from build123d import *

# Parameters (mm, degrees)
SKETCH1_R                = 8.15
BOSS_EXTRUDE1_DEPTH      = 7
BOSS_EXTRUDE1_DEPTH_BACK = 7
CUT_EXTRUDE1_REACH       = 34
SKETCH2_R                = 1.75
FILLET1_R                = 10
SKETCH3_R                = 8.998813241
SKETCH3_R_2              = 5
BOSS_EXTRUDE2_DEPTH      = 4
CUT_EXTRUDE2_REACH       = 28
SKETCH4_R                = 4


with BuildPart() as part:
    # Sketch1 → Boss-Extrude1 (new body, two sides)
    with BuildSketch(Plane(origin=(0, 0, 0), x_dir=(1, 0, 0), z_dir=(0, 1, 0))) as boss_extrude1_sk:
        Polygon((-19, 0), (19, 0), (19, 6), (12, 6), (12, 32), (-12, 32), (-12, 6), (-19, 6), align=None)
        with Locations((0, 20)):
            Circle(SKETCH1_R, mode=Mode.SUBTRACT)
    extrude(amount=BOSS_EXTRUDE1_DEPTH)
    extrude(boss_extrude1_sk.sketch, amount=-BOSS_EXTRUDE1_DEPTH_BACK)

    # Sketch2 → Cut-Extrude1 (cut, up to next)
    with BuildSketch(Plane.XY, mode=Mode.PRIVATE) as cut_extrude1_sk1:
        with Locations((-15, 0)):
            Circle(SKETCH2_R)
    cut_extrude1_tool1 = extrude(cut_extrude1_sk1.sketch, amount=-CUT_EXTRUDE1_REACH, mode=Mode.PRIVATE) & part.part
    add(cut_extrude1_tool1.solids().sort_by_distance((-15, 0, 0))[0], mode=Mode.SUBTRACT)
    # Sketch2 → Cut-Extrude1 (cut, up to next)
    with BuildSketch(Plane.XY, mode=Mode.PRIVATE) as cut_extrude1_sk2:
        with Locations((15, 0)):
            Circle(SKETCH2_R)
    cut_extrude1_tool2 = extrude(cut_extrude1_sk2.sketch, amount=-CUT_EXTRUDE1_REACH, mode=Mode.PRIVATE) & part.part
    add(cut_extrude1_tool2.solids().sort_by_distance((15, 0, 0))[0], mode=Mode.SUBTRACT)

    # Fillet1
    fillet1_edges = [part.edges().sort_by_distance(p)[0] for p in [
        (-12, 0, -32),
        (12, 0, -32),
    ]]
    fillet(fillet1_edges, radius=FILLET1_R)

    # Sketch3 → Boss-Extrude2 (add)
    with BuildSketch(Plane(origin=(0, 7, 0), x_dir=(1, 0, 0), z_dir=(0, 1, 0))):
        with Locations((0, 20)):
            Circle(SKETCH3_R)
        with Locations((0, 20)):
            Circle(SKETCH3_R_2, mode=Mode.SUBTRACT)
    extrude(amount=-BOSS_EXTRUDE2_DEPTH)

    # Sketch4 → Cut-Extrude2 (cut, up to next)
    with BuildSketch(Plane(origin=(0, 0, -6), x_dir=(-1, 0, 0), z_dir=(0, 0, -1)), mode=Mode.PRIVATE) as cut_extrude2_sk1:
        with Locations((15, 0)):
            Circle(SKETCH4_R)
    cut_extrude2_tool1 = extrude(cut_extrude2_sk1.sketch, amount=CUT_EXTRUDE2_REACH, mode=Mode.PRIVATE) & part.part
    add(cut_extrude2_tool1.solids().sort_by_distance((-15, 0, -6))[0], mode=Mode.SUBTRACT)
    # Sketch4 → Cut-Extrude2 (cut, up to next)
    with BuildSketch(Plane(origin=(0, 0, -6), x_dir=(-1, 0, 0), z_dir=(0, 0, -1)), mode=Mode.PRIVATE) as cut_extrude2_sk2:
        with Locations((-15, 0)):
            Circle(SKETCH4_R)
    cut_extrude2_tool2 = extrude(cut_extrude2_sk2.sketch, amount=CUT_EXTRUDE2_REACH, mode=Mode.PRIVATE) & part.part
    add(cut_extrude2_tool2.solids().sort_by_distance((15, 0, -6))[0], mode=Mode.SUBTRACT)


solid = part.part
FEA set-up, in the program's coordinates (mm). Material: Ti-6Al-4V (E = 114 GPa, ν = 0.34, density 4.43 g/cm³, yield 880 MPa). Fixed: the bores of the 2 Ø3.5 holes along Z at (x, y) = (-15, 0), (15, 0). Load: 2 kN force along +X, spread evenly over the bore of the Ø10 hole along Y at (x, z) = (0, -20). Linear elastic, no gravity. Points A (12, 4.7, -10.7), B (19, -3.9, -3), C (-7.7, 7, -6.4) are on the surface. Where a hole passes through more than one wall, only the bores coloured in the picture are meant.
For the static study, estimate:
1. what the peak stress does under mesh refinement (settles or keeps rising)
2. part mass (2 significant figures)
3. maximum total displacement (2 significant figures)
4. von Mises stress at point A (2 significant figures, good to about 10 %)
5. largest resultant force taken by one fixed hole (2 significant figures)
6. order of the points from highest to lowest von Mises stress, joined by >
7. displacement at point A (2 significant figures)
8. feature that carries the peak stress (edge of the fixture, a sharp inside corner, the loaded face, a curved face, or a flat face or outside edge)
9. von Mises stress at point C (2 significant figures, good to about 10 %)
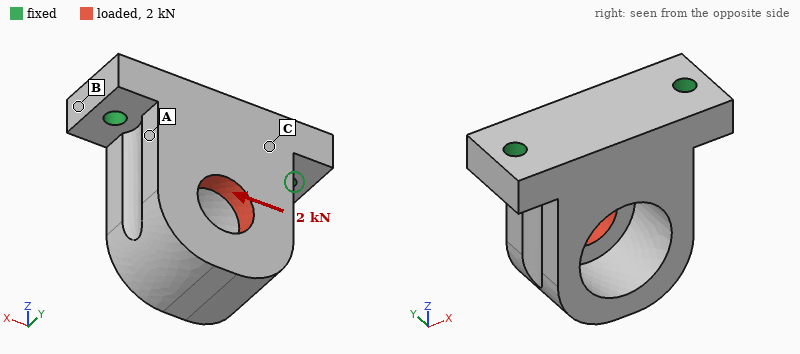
keeps rising
38 g
20 µm
35 MPa
1.7 kN
A > C > B
6.1 µm
edge of the fixture
21 MPa
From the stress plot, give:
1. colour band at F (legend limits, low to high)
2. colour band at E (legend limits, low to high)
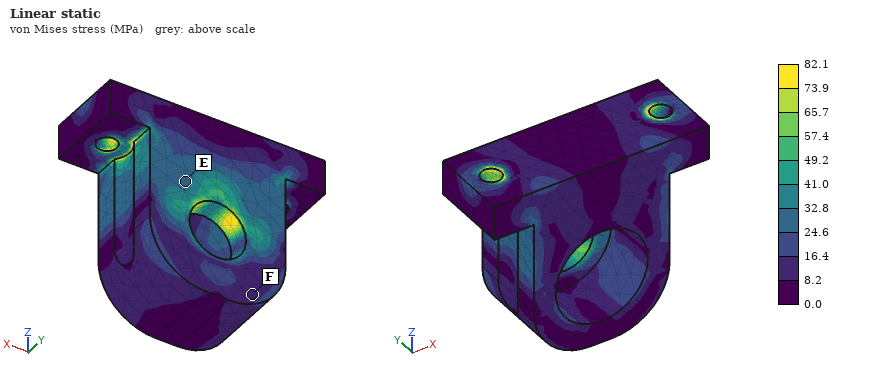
8.2 to 16.4 MPa
24.6 to 32.8 MPa
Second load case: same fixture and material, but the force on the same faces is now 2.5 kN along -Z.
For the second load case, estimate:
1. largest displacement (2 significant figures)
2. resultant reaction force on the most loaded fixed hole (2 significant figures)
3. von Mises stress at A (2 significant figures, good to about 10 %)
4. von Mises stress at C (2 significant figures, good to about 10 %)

38 µm
1.3 kN
32 MPa
24 MPa
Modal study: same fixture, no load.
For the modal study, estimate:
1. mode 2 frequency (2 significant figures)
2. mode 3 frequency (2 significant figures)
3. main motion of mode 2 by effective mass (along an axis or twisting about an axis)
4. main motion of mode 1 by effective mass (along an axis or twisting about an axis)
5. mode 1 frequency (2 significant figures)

12 kHz
20 kHz
along X
along Y
6000 Hz
